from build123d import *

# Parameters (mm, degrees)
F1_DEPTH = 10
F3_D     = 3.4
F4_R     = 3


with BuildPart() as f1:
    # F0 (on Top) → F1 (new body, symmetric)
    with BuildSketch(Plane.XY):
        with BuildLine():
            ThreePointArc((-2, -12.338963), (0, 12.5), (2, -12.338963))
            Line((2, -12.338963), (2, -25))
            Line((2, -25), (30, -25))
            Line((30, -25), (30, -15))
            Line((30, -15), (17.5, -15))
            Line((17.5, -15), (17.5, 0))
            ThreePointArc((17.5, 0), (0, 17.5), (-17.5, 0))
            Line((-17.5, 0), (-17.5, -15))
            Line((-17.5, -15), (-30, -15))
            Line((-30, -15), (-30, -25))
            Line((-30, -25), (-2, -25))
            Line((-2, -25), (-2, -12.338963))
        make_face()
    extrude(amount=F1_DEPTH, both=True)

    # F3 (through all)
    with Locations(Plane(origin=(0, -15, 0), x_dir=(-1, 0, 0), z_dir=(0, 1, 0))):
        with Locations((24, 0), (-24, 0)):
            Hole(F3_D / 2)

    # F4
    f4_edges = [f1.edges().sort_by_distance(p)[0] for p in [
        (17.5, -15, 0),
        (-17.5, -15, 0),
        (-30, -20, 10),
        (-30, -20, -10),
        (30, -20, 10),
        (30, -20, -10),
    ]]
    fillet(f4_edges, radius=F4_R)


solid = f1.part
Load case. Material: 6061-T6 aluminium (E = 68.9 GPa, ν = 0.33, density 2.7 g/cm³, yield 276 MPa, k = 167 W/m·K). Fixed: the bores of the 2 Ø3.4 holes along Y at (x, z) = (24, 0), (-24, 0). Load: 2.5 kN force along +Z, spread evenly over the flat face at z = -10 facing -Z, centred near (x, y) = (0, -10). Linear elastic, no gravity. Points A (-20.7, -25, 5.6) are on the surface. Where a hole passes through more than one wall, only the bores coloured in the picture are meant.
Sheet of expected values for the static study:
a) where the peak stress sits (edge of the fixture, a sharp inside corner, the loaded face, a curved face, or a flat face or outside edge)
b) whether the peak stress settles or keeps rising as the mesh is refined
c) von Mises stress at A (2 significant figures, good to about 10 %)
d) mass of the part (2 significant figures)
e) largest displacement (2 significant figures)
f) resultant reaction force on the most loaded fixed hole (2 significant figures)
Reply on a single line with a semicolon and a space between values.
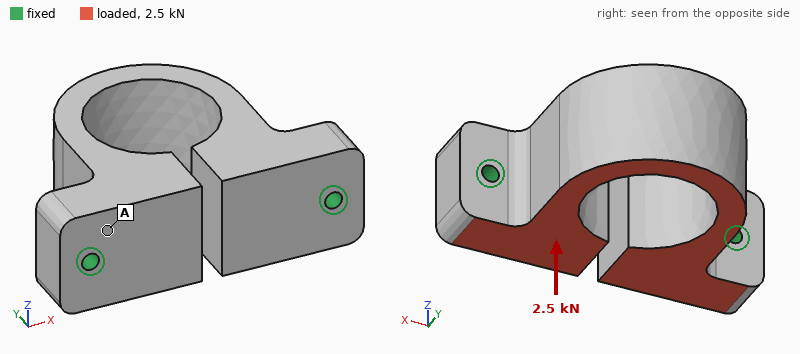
edge of the fixture; keeps rising; 21 MPa; 57 g; 73 µm; 1.3 kN
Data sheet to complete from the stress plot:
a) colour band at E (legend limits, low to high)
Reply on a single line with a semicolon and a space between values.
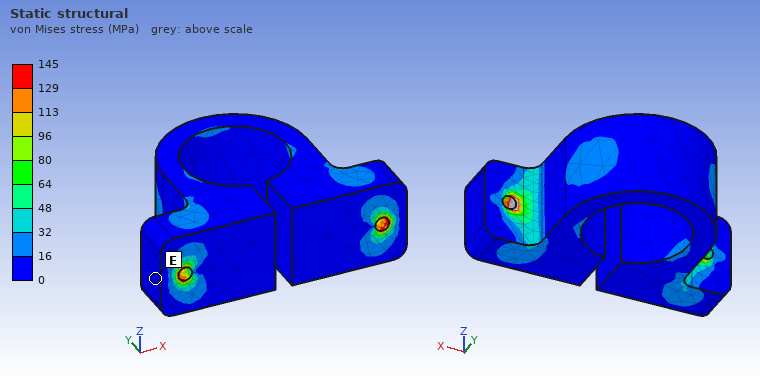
0 to 16 MPa
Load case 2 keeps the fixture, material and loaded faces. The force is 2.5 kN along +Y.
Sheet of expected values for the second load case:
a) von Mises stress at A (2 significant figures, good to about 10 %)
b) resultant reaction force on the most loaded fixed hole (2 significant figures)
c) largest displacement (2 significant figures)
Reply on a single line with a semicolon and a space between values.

22 MPa; 1.3 kN; 52 µm
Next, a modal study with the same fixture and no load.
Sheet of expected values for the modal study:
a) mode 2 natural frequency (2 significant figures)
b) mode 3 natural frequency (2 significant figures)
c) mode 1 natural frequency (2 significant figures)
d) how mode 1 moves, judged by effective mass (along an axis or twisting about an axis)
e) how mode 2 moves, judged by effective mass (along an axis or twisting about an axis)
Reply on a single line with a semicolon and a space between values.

6200 Hz; 8800 Hz; 5000 Hz; along Z; along X
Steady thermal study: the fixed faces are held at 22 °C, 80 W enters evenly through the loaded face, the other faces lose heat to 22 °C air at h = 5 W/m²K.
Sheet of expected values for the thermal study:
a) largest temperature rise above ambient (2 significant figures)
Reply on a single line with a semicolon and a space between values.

31 K
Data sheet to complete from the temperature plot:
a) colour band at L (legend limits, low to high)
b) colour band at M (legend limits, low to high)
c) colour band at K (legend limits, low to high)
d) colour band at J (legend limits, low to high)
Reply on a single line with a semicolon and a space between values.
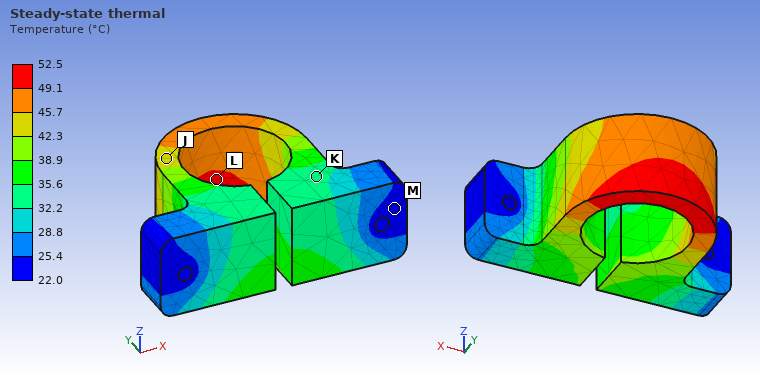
49.1 to 52.5 °C; 22.0 to 25.4 °C; 32.2 to 35.6 °C; 42.3 to 45.7 °C
